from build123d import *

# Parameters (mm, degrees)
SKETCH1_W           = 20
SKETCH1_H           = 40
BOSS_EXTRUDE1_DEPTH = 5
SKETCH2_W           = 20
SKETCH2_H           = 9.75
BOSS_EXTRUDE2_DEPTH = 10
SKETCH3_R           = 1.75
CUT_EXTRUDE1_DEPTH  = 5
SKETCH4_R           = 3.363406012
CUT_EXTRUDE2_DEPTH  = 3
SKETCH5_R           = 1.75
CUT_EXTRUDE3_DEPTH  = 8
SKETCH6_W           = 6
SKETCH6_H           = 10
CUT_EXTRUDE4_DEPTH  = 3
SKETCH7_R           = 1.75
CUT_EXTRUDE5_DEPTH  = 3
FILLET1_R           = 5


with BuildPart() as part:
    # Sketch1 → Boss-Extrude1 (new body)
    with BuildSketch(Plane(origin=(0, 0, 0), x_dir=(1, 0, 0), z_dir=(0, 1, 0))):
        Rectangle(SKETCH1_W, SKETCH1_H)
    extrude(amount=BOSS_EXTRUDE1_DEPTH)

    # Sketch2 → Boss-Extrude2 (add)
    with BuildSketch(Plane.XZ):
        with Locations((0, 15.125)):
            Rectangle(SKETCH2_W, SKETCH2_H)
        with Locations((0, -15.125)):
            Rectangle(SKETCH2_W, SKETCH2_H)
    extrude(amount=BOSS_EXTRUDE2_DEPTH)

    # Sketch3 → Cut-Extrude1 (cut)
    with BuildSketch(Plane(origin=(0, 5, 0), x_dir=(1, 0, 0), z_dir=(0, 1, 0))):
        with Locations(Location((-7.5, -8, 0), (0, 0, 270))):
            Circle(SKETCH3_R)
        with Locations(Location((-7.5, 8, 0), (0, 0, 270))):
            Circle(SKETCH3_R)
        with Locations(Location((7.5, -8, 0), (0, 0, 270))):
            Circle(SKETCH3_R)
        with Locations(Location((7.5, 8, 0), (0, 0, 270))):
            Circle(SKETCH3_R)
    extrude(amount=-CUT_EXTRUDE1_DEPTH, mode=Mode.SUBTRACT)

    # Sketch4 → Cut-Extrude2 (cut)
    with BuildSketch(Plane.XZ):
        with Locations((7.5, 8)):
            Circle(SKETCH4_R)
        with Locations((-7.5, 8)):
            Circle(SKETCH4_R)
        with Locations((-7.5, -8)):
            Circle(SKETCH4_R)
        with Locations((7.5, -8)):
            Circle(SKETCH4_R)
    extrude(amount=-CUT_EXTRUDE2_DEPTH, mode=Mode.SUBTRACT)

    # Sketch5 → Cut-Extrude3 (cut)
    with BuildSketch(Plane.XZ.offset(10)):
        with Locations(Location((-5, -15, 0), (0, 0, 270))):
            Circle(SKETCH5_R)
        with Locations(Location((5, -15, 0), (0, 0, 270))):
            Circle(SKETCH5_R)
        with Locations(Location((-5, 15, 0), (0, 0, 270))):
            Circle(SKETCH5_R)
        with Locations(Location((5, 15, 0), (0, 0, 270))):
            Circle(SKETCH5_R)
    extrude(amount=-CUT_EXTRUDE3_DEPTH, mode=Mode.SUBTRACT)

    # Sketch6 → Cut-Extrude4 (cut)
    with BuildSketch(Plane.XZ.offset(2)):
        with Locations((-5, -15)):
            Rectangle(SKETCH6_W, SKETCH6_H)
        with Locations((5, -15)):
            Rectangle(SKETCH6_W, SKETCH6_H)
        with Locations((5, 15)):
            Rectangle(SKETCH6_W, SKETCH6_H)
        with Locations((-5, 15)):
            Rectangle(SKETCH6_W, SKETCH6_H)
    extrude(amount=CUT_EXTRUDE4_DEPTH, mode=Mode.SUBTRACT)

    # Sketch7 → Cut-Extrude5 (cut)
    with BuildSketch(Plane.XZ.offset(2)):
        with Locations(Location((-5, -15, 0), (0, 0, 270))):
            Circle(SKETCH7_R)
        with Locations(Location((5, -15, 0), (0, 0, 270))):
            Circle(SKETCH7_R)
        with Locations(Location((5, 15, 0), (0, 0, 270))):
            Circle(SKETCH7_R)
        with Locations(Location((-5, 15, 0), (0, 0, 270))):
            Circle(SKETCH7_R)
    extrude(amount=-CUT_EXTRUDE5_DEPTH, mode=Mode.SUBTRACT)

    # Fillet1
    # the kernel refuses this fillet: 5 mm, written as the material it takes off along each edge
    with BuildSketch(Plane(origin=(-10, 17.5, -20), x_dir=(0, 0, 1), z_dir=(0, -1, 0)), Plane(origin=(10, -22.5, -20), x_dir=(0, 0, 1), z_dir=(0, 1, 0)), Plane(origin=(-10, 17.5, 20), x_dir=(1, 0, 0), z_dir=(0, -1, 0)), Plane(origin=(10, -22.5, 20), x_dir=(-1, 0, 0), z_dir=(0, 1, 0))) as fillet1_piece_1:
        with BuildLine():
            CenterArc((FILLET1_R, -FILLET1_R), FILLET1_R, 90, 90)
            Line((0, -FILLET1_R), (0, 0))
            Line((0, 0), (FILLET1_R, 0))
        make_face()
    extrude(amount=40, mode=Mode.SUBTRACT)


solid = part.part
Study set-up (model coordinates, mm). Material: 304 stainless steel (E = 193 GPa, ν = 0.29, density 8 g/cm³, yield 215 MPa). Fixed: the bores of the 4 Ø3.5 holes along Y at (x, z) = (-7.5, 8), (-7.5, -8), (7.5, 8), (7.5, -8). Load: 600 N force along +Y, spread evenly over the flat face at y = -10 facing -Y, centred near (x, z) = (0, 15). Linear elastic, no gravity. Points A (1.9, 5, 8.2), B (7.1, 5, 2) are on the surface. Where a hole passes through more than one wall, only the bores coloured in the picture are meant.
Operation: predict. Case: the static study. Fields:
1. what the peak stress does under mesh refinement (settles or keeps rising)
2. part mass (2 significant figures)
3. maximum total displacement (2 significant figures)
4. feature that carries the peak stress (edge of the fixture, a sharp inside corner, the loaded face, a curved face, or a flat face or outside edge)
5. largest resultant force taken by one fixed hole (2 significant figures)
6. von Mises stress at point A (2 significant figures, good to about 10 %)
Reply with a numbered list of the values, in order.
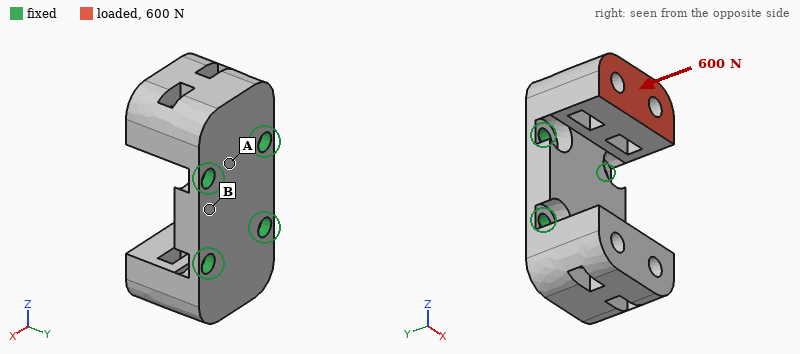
1. keeps rising
2. 49 g
3. 14 µm
4. edge of the fixture
5. 420 N
6. 31 MPa
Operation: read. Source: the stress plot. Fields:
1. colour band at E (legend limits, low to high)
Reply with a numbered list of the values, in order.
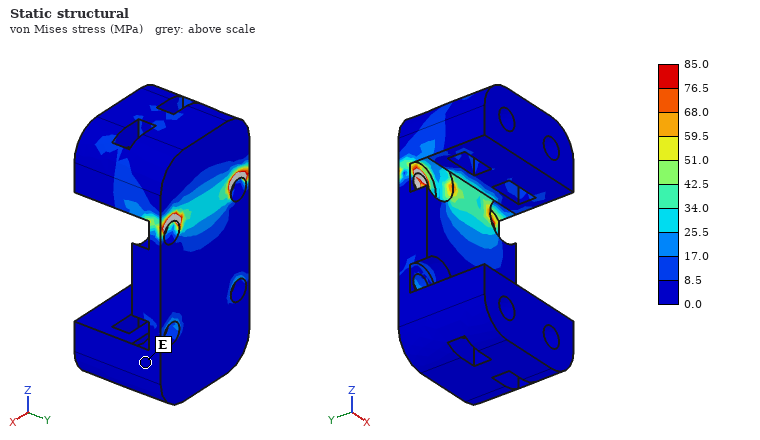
1. 0.0 to 8.5 MPa
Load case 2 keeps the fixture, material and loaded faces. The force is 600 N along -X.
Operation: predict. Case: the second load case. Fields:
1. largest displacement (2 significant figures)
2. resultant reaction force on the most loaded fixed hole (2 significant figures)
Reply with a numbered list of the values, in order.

1. 9.5 µm
2. 680 N
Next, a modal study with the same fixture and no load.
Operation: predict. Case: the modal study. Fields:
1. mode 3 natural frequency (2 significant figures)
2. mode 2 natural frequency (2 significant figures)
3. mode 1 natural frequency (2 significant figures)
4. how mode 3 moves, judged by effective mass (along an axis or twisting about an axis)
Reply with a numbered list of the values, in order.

1. 16 kHz
2. 7900 Hz
3. 7700 Hz
4. along X
